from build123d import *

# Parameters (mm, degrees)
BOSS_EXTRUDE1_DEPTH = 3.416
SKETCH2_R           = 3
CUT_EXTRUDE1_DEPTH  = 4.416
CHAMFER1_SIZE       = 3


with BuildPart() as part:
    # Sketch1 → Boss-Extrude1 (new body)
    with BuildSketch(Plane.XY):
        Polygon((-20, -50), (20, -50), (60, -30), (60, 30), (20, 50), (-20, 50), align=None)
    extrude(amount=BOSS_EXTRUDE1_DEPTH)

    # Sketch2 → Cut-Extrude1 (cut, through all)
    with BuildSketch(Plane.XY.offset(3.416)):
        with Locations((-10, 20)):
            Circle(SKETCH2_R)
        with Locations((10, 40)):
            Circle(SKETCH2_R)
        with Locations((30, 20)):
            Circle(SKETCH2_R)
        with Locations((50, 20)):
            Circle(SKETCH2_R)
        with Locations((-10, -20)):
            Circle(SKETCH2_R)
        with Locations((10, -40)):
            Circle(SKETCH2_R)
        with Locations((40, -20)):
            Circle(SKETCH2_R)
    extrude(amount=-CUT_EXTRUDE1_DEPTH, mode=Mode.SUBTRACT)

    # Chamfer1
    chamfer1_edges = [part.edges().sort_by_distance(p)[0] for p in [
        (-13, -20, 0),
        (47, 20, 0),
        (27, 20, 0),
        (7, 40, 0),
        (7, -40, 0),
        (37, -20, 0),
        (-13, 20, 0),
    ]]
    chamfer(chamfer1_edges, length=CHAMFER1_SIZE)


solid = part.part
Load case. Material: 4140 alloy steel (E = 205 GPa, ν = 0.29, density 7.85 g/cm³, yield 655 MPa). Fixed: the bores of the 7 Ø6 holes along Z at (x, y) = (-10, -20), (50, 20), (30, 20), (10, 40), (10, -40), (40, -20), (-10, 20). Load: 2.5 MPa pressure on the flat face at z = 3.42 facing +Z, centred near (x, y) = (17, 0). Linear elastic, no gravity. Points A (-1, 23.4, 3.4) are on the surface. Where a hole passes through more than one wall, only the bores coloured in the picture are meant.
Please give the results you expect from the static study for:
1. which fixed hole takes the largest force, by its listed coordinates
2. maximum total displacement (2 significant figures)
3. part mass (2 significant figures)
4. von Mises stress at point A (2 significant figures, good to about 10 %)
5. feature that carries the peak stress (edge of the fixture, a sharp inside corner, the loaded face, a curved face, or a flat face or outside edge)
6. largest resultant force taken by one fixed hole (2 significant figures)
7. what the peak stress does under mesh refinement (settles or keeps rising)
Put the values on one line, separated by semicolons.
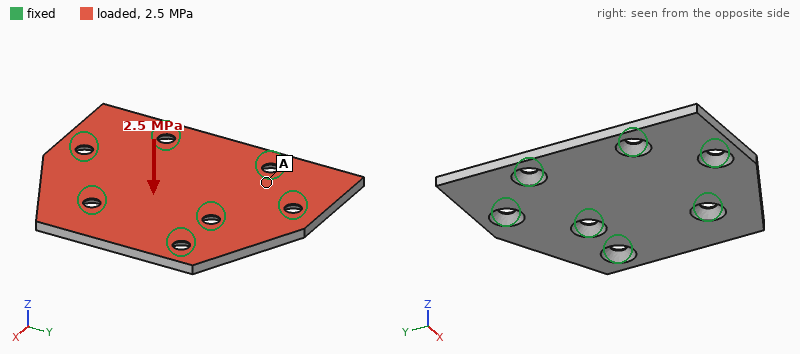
(40, -20); 0.16 mm; 180 g; 120 MPa; edge of the fixture; 3.7 kN; keeps rising
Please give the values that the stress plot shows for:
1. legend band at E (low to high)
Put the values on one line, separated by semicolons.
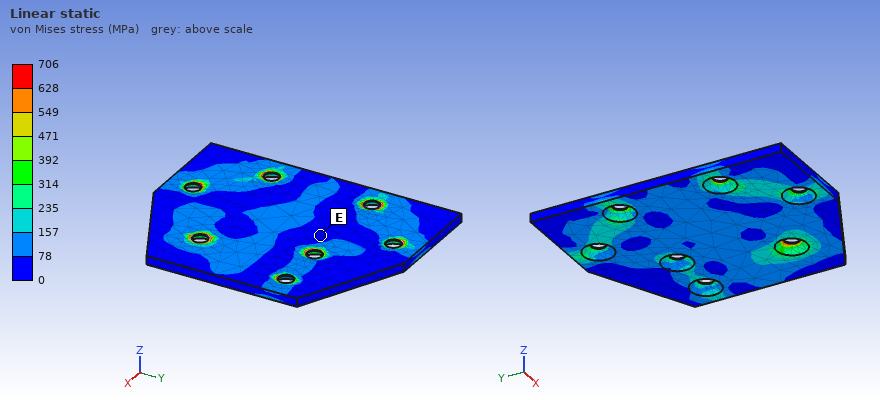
0 to 78 MPa
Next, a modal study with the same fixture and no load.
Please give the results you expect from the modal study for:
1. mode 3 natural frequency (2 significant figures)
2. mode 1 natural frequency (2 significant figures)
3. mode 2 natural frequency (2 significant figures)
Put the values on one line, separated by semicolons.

5700 Hz; 4700 Hz; 4800 Hz
